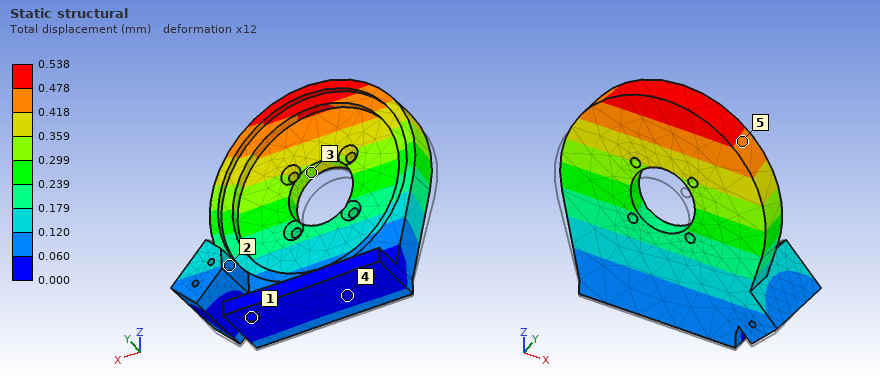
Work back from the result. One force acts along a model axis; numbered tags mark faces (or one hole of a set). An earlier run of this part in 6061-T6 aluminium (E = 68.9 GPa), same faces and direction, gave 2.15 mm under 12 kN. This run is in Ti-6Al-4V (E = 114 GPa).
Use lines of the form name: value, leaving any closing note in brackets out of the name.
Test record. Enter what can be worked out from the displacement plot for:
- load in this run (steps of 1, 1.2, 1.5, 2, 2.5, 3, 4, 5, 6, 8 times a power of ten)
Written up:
load in this run: 5 kN
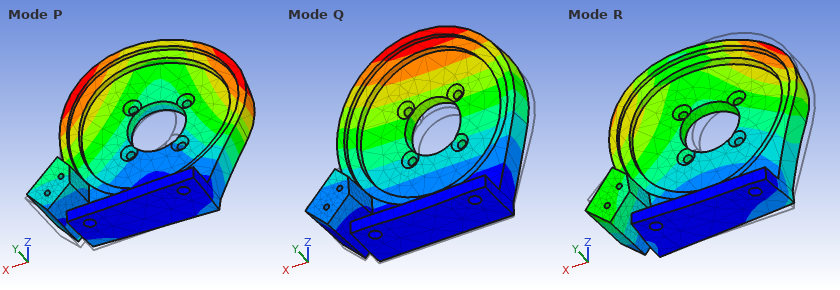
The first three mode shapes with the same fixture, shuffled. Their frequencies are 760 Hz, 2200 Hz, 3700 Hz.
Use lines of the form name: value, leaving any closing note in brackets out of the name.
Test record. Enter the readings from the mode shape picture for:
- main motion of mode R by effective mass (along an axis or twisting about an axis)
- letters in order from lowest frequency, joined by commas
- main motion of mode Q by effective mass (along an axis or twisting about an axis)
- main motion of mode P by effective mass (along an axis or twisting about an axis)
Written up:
main motion of mode R by effective mass: along X
letters in order from lowest frequency, joined by commas: Q, P, R
main motion of mode Q by effective mass: along Y
main motion of mode P by effective mass: along X
